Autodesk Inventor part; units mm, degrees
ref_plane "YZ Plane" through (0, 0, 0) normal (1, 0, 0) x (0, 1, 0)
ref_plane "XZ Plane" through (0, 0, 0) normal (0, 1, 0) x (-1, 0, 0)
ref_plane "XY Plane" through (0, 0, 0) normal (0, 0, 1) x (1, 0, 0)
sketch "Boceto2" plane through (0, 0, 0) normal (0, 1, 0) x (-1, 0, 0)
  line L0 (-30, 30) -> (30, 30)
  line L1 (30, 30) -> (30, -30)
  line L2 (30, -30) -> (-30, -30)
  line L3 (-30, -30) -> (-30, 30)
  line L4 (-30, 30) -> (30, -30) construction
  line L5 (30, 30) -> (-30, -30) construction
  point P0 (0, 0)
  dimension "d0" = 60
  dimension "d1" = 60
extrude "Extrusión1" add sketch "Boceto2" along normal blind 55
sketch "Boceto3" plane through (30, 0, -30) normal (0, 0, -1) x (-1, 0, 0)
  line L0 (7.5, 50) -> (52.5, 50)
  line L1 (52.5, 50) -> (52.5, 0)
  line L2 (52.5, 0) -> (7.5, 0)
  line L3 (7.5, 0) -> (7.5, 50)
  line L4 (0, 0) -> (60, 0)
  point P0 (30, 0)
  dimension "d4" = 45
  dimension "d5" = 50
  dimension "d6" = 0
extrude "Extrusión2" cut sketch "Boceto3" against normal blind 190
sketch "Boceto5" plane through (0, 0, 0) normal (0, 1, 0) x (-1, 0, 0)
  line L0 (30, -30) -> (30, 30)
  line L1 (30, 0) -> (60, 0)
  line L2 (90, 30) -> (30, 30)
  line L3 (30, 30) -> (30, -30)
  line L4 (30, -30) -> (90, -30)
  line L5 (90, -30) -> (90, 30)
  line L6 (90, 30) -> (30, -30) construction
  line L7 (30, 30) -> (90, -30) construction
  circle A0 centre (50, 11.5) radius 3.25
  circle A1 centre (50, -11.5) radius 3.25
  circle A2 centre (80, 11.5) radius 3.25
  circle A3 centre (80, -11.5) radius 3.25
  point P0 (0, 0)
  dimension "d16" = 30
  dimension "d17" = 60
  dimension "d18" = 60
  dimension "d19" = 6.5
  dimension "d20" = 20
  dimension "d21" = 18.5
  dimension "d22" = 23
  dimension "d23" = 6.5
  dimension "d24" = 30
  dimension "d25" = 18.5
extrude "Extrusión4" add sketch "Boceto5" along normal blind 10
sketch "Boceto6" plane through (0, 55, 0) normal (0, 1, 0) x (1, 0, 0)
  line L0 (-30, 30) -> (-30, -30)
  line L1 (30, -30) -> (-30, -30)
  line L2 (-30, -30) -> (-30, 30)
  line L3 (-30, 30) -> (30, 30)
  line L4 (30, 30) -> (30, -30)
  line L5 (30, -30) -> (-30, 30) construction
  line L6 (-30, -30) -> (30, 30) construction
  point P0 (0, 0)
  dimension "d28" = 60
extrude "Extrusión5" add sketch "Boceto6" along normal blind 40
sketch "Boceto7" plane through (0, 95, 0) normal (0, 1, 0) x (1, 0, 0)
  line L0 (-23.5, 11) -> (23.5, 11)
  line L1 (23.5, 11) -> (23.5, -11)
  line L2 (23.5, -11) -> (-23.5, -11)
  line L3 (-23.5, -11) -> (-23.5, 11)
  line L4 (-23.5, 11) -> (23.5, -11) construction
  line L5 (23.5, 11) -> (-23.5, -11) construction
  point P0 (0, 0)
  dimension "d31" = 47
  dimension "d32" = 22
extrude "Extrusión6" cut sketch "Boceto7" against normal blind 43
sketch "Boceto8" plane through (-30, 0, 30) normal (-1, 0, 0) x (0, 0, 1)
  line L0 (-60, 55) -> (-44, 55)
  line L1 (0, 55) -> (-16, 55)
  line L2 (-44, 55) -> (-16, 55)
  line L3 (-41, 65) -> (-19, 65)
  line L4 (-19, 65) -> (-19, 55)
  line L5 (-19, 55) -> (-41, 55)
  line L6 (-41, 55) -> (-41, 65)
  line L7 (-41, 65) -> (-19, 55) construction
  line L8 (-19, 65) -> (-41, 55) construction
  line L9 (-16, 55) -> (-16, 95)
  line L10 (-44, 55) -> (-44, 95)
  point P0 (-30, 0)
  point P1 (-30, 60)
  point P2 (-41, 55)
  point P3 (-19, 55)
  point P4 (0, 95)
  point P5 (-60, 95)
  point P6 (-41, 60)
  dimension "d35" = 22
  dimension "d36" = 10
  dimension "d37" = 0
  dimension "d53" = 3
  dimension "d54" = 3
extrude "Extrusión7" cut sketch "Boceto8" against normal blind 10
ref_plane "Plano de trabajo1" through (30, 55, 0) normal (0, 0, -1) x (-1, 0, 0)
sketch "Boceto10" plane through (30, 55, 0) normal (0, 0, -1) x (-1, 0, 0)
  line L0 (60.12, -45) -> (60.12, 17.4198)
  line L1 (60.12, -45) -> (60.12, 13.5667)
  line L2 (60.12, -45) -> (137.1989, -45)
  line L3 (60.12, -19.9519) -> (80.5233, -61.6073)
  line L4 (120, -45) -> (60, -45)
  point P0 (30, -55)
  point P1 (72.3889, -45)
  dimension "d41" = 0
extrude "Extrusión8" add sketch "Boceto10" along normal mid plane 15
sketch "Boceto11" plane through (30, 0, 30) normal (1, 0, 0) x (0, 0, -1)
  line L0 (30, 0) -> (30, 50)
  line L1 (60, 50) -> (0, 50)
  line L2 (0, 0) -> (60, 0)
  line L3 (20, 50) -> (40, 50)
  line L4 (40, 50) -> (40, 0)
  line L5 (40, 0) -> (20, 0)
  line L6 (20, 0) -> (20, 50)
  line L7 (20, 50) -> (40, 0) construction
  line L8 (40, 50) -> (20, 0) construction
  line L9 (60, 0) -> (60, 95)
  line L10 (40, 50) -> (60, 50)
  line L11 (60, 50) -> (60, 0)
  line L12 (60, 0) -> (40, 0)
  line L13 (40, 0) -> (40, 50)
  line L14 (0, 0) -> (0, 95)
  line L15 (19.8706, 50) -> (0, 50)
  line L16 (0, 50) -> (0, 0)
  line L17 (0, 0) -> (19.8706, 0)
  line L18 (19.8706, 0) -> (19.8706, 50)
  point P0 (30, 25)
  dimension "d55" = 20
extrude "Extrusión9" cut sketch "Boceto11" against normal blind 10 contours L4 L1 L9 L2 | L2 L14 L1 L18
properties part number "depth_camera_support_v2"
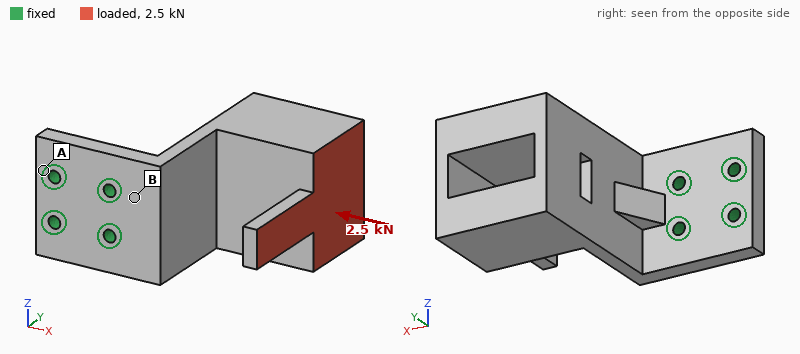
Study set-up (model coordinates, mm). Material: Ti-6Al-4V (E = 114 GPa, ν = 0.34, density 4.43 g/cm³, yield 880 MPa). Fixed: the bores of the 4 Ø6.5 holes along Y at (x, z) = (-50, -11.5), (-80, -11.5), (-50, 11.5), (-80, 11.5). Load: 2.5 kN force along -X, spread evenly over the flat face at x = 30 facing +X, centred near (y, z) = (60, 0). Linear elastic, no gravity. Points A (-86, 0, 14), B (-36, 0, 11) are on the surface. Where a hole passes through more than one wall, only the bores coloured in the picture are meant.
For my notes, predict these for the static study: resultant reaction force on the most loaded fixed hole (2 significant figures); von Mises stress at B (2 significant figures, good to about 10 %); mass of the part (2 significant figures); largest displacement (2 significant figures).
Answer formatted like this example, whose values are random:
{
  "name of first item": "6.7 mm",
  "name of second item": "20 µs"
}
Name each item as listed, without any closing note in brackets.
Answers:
{
  "resultant reaction force on the most loaded fixed hole": "1.4 kN",
  "von Mises stress at B": "110 MPa",
  "mass of the part": "810 g",
  "largest displacement": "1.8 mm"
}
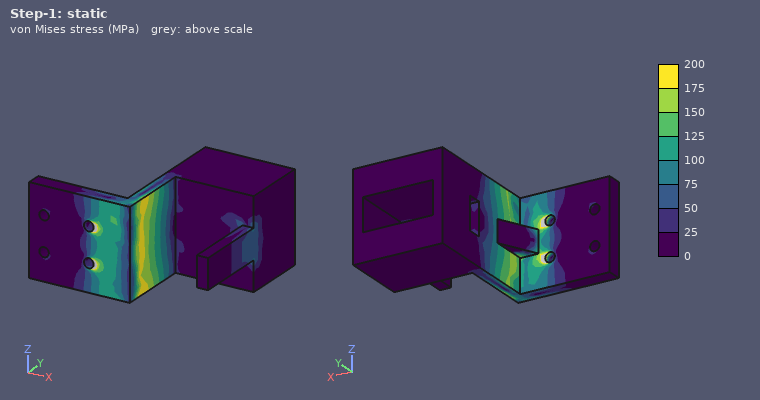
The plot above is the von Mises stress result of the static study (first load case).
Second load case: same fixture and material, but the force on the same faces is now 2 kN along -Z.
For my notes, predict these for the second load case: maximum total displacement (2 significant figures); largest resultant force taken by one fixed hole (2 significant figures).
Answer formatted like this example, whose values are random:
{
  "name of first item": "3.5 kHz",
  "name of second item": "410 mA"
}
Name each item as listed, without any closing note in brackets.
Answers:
{
  "maximum total displacement": "0.56 mm",
  "largest resultant force taken by one fixed hole": "5.1 kN"
}
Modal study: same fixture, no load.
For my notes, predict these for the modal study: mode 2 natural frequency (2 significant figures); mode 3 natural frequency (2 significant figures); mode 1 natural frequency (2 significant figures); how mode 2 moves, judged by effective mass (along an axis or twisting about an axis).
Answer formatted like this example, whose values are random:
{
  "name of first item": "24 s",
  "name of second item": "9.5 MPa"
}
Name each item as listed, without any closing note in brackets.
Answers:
{
  "mode 2 natural frequency": "600 Hz",
  "mode 3 natural frequency": "1000 Hz",
  "mode 1 natural frequency": "240 Hz",
  "how mode 2 moves, judged by effective mass": "along Z"
}
